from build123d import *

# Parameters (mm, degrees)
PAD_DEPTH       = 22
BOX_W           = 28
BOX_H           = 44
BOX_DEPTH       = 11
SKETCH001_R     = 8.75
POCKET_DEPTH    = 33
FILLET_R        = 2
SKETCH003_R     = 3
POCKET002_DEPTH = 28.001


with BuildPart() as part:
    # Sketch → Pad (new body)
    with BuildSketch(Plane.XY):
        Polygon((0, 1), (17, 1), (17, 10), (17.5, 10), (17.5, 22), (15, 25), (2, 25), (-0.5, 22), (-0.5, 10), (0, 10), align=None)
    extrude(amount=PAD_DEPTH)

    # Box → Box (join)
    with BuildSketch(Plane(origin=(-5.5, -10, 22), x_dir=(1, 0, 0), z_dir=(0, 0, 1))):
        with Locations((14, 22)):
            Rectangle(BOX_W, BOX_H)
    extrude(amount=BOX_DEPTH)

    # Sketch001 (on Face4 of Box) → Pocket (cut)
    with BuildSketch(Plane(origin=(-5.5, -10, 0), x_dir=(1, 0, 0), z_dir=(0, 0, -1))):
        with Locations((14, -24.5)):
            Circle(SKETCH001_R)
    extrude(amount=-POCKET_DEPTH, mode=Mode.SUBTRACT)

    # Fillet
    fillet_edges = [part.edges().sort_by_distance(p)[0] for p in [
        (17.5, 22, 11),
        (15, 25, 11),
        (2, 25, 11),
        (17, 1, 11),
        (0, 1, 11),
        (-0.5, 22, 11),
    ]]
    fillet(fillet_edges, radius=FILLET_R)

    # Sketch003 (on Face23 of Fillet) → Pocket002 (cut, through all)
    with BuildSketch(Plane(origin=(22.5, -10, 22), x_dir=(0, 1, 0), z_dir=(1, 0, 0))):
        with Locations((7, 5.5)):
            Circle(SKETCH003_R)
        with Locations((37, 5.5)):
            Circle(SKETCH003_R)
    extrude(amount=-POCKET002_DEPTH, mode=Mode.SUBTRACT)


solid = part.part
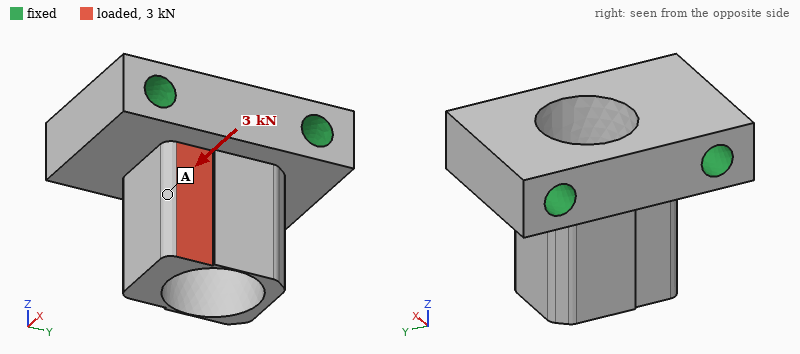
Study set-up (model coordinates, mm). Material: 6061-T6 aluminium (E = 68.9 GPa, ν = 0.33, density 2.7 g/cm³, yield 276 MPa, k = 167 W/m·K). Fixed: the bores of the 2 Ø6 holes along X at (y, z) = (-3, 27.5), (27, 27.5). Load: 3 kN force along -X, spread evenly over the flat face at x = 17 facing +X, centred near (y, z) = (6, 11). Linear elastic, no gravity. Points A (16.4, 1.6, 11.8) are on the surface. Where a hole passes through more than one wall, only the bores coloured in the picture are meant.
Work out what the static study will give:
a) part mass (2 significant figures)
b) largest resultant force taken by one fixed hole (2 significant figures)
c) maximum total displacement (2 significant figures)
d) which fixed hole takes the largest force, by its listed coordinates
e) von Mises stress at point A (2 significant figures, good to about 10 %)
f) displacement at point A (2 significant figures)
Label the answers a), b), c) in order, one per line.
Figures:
a) 35 g
b) 2.7 kN
c) 92 µm
d) (-3, 27.5)
e) 26 MPa
f) 33 µm
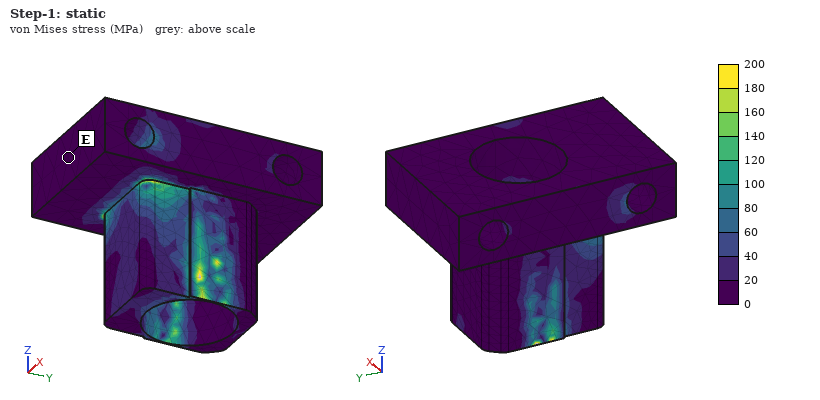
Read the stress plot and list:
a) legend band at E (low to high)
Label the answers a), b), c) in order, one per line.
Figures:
a) 0 to 20 MPa
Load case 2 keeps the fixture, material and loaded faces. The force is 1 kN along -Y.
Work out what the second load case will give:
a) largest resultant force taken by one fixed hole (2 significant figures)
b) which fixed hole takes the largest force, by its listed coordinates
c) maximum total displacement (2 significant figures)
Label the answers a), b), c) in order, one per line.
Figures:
a) 850 N
b) (-3, 27.5)
c) 34 µm
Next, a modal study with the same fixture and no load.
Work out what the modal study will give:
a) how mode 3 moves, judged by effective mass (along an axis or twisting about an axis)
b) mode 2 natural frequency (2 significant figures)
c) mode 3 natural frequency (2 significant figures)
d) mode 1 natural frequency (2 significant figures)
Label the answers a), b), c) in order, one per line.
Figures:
a) along X
b) 16 kHz
c) 17 kHz
d) 16 kHz
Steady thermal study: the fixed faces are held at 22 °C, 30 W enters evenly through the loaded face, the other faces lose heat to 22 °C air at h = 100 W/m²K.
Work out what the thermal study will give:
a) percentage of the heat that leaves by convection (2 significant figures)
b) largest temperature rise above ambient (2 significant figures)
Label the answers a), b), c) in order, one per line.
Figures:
a) 9.5 %
b) 26 K
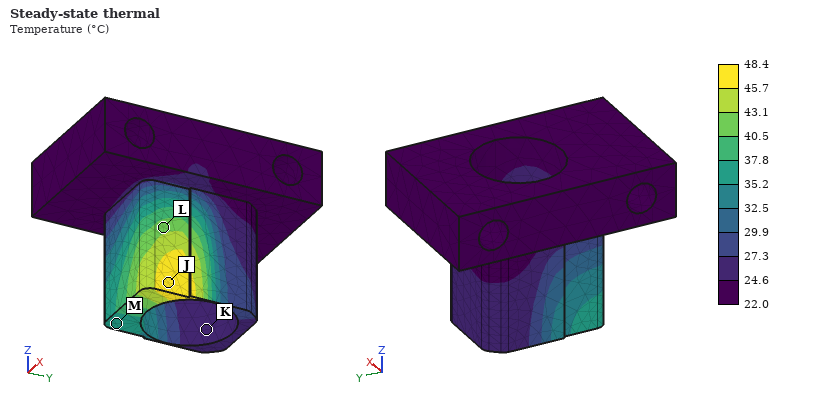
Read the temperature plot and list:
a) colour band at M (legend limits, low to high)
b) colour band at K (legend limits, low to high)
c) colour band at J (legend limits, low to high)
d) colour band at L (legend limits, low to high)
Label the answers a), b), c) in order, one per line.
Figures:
a) 35.2 to 37.8 °C
b) 24.6 to 27.3 °C
c) 45.7 to 48.4 °C
d) 40.5 to 43.1 °C
